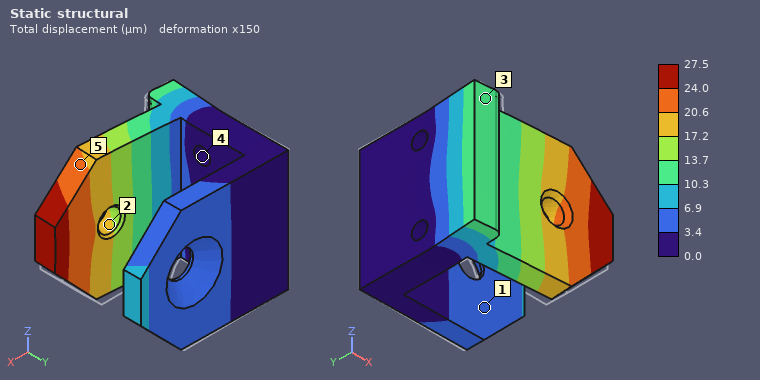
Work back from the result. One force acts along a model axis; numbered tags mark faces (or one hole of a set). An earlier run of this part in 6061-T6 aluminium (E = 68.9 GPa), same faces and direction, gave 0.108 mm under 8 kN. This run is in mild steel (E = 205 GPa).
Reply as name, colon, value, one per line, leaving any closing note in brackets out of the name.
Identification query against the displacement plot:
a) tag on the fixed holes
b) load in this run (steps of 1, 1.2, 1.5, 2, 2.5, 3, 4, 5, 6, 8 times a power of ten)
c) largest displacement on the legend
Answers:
tag on the fixed holes: 4
load in this run: 6 kN
largest displacement on the legend: 27.5 µm
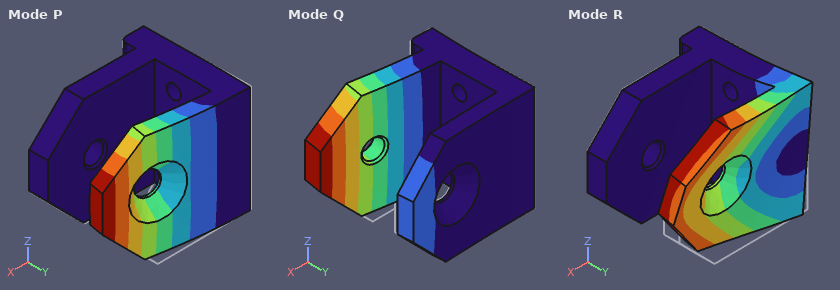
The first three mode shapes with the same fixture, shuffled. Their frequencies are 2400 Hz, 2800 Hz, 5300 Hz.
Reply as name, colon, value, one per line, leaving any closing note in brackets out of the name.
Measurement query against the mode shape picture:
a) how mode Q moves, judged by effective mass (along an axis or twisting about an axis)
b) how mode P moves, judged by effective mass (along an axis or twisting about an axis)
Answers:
how mode Q moves, judged by effective mass: along Y
how mode P moves, judged by effective mass: along Y
